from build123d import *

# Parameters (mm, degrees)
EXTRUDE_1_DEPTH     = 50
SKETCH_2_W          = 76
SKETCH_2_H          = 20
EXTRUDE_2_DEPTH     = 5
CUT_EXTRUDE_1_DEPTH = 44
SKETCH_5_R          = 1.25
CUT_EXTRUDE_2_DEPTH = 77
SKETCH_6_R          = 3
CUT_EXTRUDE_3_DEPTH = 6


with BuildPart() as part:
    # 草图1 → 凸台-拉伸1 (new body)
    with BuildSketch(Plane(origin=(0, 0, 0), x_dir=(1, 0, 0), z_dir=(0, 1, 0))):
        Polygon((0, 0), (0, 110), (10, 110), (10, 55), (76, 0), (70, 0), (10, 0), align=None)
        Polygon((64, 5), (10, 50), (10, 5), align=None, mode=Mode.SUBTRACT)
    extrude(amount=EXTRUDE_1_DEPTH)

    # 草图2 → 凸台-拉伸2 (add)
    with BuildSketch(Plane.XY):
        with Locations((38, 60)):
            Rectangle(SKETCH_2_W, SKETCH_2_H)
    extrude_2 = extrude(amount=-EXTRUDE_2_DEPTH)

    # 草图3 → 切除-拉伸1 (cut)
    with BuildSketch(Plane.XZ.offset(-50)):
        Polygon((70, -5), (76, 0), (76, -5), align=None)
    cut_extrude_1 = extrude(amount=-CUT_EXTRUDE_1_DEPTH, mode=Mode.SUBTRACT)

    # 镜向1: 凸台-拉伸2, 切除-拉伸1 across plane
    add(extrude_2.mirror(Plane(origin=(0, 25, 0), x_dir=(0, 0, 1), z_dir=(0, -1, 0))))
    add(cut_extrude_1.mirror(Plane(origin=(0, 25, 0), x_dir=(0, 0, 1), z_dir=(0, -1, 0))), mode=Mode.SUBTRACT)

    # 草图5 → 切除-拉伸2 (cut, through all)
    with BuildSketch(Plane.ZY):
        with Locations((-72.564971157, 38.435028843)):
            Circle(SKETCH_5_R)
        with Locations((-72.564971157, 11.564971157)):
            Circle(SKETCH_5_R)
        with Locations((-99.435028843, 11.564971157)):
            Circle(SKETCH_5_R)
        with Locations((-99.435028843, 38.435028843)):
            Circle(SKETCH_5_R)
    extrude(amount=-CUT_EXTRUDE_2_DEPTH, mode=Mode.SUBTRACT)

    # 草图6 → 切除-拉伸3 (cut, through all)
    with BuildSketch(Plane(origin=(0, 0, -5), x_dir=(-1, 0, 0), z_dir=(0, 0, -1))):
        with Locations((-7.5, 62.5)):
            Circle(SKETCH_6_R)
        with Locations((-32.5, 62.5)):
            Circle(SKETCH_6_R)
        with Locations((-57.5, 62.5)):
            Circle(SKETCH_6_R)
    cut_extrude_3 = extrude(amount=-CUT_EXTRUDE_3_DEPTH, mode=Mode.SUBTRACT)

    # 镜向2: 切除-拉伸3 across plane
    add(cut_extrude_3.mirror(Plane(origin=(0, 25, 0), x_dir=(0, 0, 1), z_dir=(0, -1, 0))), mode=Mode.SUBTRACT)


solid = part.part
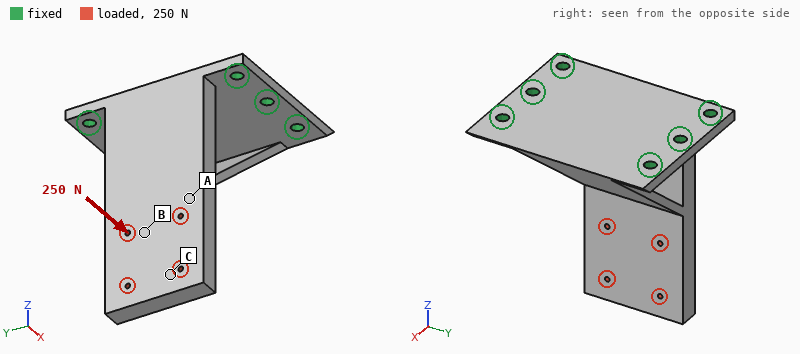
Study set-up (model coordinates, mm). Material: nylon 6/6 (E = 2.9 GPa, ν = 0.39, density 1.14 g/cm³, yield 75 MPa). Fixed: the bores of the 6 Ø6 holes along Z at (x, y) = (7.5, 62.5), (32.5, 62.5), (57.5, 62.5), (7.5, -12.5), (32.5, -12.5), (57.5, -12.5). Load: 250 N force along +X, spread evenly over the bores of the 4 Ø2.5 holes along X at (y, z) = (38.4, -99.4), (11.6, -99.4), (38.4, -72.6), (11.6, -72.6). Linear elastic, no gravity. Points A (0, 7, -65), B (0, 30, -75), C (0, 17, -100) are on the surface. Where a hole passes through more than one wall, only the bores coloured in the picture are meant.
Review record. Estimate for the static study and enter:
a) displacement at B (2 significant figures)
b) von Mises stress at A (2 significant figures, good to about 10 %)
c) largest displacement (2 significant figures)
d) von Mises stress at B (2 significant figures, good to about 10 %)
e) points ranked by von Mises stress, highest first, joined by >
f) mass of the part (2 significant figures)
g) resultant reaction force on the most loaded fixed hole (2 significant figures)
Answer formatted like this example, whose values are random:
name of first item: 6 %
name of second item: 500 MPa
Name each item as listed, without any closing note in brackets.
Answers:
displacement at B: 0.95 mm
von Mises stress at A: 6.1 MPa
largest displacement: 1.9 mm
von Mises stress at B: 3.6 MPa
points ranked by von Mises stress, highest first, joined by >: A > B > C
mass of the part: 110 g
resultant reaction force on the most loaded fixed hole: 220 N
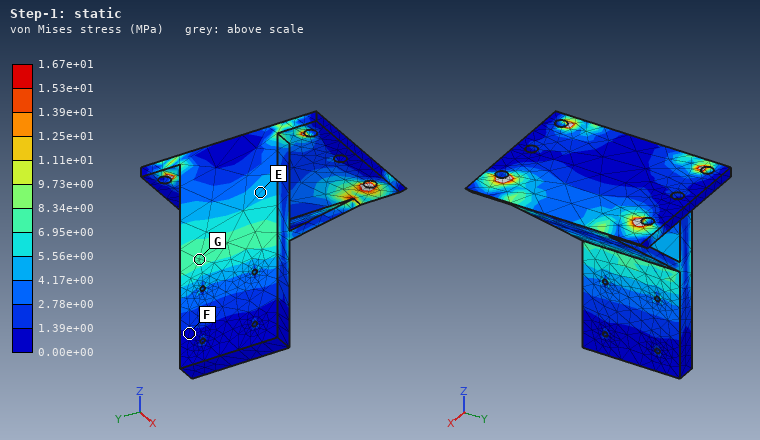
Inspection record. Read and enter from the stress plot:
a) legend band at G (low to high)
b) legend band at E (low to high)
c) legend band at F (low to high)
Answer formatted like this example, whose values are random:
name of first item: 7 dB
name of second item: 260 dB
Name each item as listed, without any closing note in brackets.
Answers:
legend band at G: 6.95e+00 to 8.34e+00 MPa
legend band at E: 4.17e+00 to 5.56e+00 MPa
legend band at F: 0.00e+00 to 1.39e+00 MPa
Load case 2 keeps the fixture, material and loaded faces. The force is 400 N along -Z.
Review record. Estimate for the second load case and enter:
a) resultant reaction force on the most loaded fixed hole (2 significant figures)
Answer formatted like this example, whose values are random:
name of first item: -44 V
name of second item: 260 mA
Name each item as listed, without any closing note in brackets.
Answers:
resultant reaction force on the most loaded fixed hole: 220 N
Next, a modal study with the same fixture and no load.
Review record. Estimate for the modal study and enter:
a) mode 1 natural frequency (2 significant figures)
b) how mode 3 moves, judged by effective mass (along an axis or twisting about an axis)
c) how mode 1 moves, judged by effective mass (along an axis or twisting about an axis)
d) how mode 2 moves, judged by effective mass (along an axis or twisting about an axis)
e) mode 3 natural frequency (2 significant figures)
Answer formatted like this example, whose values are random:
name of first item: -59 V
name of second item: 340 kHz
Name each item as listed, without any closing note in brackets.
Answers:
mode 1 natural frequency: 390 Hz
how mode 3 moves, judged by effective mass: along Z
how mode 1 moves, judged by effective mass: along X
how mode 2 moves, judged by effective mass: along Y
mode 3 natural frequency: 880 Hz
